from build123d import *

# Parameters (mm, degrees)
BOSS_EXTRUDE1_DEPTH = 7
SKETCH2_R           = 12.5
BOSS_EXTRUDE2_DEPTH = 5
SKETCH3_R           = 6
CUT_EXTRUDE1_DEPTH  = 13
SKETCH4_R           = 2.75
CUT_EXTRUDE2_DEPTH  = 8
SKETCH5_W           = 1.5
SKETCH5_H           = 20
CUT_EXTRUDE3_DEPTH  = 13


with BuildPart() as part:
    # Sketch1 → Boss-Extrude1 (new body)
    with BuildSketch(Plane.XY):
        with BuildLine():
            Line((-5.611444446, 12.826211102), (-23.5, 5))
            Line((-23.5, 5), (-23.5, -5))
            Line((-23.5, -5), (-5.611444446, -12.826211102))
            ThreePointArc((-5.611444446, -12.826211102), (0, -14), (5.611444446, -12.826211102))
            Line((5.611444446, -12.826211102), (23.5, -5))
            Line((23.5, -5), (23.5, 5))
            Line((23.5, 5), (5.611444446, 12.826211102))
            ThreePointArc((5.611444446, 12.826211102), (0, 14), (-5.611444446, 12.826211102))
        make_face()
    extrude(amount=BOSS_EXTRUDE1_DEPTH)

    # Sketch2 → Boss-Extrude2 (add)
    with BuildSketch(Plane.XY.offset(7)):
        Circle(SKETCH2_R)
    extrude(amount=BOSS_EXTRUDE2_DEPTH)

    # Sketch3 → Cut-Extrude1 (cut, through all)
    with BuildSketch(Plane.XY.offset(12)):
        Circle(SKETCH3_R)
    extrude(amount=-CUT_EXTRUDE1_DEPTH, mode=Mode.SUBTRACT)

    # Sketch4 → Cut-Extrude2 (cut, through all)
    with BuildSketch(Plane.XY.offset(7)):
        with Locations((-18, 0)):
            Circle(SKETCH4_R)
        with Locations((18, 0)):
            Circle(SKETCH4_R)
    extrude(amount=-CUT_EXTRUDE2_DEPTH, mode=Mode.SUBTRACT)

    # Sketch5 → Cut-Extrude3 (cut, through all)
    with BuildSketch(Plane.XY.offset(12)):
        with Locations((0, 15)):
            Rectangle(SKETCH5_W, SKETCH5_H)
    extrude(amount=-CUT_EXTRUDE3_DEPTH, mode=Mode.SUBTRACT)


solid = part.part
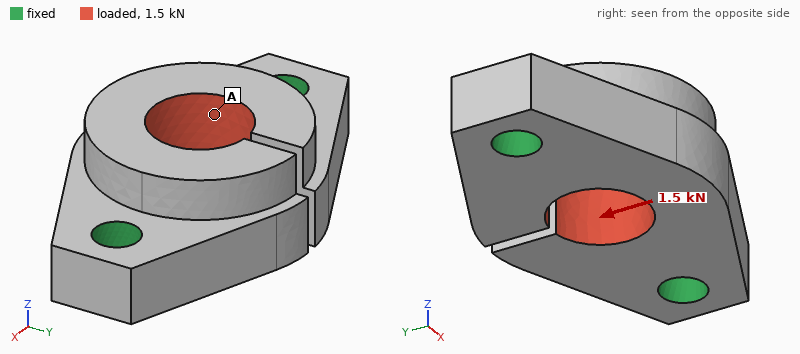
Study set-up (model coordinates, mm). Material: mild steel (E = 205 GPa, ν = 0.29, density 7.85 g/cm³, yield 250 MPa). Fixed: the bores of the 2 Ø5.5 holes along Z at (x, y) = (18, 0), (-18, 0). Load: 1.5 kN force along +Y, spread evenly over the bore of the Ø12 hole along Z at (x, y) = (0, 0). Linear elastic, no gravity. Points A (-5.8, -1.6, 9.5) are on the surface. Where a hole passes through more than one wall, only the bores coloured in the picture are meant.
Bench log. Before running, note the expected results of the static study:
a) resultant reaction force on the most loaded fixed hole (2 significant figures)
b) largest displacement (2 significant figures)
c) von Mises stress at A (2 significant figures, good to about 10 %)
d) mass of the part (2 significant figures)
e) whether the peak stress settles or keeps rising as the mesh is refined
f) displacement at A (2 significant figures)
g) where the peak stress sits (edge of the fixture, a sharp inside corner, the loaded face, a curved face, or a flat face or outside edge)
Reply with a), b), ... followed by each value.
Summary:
a) 940 N
b) 4.4 µm
c) 8.7 MPa
d) 57 g
e) keeps rising
f) 2.2 µm
g) edge of the fixture
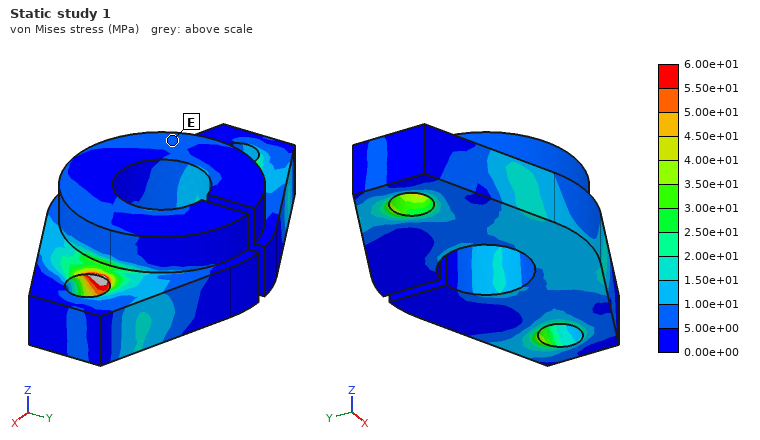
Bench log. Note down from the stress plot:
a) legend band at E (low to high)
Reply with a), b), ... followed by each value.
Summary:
a) 5.00e+00 to 1.00e+01 MPa
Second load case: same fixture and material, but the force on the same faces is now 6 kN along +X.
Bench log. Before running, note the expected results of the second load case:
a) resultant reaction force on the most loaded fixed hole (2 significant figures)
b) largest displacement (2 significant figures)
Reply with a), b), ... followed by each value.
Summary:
a) 3.0 kN
b) 6.3 µm
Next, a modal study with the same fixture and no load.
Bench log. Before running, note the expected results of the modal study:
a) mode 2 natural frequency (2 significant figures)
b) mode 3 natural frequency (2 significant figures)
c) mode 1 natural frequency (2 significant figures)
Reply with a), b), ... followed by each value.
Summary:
a) 17 kHz
b) 17 kHz
c) 16 kHz
